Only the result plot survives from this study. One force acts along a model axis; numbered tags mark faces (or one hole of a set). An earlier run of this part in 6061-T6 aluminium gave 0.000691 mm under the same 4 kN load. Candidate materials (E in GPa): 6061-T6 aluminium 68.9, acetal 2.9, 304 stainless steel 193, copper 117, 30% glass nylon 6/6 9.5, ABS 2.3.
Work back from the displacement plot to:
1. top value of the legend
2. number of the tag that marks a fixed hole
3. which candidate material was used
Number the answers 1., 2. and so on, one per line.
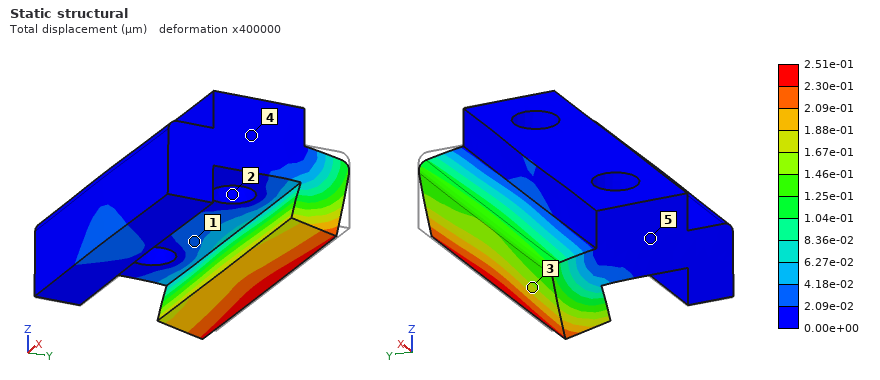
1. 2.51e-01 µm
2. 2
3. 304 stainless steel
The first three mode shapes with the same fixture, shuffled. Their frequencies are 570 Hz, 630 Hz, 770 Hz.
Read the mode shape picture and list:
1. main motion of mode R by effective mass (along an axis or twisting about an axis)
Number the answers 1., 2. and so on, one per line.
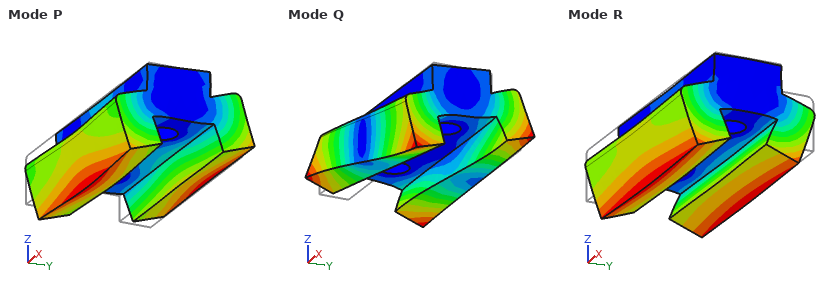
1. along Z
